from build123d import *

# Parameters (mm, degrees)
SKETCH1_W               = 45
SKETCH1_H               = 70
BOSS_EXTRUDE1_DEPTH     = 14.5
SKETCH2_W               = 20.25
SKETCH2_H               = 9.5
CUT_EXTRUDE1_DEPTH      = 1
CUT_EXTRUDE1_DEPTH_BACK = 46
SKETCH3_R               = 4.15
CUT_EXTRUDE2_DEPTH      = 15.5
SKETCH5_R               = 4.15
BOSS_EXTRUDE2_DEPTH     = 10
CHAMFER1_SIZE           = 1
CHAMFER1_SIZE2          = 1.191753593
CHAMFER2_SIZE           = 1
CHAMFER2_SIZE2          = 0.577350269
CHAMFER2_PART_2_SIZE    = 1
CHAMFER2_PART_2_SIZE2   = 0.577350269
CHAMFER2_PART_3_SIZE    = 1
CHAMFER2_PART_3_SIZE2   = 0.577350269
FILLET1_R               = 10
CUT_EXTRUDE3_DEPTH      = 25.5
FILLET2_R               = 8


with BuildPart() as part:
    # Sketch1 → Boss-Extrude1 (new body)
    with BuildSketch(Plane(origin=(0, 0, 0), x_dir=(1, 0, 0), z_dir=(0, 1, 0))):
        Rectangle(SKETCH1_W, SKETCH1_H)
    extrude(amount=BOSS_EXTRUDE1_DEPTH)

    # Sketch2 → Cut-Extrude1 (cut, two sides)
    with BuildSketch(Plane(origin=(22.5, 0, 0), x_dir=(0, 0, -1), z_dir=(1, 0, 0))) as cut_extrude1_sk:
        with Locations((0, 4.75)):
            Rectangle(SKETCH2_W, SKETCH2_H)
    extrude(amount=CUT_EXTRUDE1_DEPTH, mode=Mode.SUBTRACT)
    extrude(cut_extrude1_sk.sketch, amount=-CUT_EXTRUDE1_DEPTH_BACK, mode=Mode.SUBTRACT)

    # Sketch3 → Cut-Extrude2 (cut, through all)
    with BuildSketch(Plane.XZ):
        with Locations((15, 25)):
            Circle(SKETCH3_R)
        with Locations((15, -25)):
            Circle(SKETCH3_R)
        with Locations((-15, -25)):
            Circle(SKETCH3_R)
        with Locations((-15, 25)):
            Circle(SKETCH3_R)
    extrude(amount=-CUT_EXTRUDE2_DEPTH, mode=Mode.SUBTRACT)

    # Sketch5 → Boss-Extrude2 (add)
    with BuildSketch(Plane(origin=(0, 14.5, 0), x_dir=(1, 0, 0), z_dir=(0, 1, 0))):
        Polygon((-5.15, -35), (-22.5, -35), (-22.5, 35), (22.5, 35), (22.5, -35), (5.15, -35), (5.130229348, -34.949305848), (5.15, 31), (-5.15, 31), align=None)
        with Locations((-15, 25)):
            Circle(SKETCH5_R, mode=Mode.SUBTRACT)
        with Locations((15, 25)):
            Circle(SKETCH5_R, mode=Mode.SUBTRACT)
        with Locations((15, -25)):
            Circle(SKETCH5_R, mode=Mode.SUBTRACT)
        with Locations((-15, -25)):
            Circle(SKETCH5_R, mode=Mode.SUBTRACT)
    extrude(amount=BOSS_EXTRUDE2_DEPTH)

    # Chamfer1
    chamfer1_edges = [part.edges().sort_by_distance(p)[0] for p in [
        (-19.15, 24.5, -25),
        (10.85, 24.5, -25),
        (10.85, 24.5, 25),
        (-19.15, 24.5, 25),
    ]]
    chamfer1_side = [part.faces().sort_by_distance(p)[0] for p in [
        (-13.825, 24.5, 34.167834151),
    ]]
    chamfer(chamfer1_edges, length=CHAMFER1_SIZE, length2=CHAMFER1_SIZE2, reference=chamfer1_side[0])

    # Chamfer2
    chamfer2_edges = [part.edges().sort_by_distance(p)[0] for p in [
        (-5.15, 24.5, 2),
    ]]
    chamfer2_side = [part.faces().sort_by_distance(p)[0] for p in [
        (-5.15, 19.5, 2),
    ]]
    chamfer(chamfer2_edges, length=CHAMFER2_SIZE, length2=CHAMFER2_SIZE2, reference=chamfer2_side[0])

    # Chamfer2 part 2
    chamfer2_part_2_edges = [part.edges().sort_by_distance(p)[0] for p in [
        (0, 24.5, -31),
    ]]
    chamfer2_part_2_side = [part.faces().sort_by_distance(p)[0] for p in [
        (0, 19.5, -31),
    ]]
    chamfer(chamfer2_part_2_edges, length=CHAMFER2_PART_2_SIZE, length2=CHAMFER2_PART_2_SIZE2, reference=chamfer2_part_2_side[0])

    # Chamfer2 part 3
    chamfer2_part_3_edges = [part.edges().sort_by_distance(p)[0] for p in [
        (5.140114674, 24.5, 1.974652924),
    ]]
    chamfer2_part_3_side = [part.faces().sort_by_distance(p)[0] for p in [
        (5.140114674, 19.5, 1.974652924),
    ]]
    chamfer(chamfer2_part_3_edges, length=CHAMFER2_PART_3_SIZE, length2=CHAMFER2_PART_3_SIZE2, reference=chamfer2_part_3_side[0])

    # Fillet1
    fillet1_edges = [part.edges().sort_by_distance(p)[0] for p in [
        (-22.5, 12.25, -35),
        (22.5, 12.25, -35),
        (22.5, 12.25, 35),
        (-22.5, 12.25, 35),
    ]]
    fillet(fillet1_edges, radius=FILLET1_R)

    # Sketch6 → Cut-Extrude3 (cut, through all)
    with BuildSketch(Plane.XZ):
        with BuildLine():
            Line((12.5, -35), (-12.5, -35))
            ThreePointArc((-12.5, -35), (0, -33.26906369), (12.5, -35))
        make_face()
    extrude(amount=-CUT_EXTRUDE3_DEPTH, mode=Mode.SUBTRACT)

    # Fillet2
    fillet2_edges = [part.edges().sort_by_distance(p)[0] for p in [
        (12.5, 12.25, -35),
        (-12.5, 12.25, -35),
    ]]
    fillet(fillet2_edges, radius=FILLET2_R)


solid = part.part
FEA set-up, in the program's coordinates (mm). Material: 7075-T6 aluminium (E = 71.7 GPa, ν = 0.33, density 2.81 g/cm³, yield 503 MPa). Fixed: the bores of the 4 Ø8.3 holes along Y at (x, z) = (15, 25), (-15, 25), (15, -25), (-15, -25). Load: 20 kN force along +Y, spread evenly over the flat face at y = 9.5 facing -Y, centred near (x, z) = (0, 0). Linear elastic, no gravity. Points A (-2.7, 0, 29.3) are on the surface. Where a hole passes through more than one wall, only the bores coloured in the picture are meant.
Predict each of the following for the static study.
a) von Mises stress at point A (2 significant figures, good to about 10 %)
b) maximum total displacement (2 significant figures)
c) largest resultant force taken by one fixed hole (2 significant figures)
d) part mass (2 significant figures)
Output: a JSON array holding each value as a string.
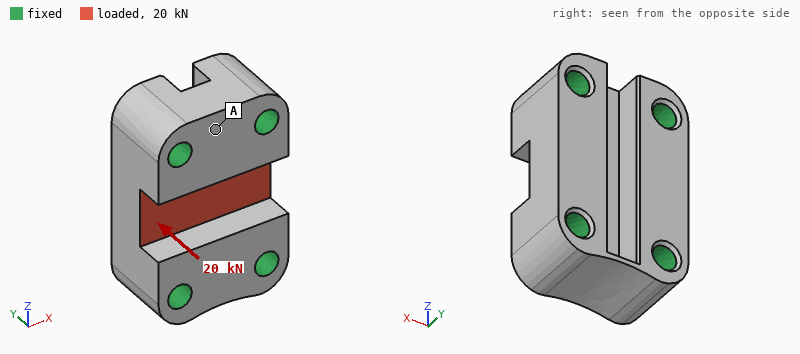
["8.4 MPa", "23 µm", "5.1 kN", "150 g"]
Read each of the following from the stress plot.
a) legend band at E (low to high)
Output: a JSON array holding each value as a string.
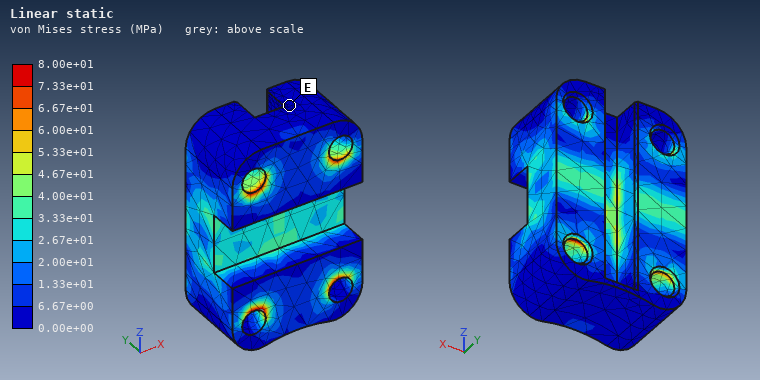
["0.00e+00 to 6.67e+00 MPa"]
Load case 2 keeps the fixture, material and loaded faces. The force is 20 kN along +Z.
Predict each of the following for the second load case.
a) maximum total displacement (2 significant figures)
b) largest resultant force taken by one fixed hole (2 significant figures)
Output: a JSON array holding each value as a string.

["9.2 µm", "5.2 kN"]
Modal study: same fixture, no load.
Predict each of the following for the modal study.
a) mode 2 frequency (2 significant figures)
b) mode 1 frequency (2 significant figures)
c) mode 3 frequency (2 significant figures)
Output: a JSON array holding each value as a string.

["29 kHz", "28 kHz", "32 kHz"]
